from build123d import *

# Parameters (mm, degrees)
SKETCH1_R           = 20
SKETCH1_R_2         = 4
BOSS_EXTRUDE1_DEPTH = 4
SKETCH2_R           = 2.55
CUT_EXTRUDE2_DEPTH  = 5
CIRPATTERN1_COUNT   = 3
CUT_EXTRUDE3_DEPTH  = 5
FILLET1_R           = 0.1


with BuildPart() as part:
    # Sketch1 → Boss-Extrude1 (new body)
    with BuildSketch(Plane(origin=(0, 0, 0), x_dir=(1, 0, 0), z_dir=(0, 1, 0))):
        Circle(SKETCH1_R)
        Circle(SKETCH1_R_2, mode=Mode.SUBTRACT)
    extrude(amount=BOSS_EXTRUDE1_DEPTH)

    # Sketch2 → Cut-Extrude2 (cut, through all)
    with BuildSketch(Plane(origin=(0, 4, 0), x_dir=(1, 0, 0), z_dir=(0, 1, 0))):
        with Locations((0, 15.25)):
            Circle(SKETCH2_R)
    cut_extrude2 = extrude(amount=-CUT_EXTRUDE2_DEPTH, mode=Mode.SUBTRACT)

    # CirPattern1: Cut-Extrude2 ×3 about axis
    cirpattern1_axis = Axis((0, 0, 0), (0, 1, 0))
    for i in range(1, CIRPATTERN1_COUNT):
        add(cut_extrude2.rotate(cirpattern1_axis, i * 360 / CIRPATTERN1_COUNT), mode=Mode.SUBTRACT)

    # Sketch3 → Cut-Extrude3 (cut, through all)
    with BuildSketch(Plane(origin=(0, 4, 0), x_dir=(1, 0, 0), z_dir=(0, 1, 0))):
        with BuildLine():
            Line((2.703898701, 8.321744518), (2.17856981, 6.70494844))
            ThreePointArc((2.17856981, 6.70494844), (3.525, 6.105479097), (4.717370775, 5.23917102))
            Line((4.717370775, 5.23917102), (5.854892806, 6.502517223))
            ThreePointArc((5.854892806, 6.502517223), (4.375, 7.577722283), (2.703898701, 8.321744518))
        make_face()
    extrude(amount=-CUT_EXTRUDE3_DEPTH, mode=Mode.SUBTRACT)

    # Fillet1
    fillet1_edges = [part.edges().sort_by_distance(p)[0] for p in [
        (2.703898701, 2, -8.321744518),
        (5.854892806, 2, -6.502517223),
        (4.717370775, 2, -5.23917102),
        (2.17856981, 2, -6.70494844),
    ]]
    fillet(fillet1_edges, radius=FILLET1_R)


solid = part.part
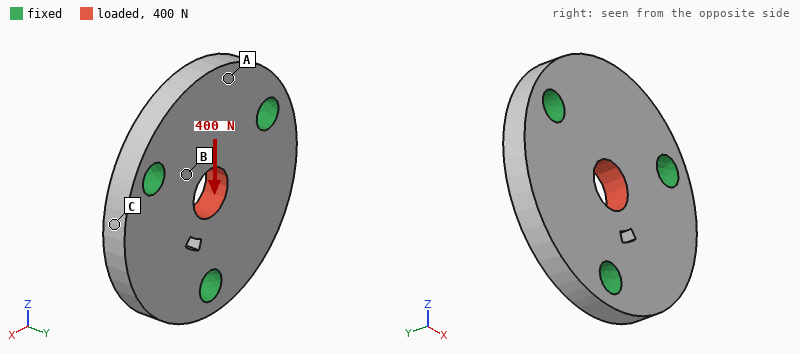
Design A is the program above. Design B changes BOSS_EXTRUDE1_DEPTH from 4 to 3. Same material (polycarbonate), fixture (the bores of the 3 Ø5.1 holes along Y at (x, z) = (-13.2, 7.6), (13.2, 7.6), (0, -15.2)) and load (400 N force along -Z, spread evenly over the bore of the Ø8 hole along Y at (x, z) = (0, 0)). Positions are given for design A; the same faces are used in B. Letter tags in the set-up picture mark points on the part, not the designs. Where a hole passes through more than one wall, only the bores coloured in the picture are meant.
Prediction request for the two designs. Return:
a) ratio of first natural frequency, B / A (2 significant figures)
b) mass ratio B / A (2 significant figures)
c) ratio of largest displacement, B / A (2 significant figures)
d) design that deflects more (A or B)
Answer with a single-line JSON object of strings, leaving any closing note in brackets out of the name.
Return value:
{"ratio of first natural frequency, B / A": "0.80", "mass ratio B / A": "0.75", "ratio of largest displacement, B / A": "1.3", "design that deflects more": "B"}
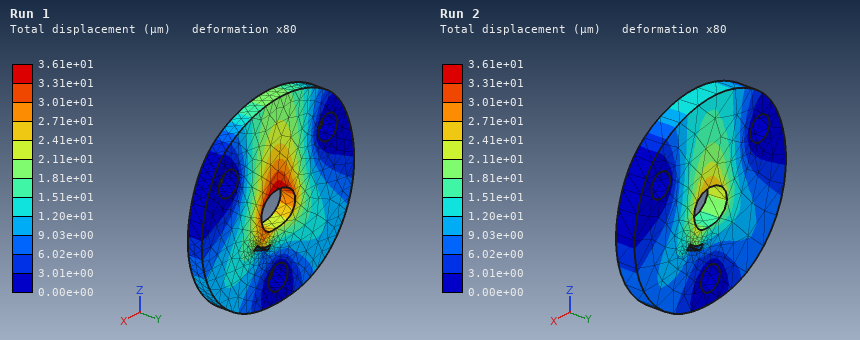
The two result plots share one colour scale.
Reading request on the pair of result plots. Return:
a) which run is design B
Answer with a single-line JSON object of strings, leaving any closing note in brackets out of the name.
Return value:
{"which run is design B": "Run 1"}
